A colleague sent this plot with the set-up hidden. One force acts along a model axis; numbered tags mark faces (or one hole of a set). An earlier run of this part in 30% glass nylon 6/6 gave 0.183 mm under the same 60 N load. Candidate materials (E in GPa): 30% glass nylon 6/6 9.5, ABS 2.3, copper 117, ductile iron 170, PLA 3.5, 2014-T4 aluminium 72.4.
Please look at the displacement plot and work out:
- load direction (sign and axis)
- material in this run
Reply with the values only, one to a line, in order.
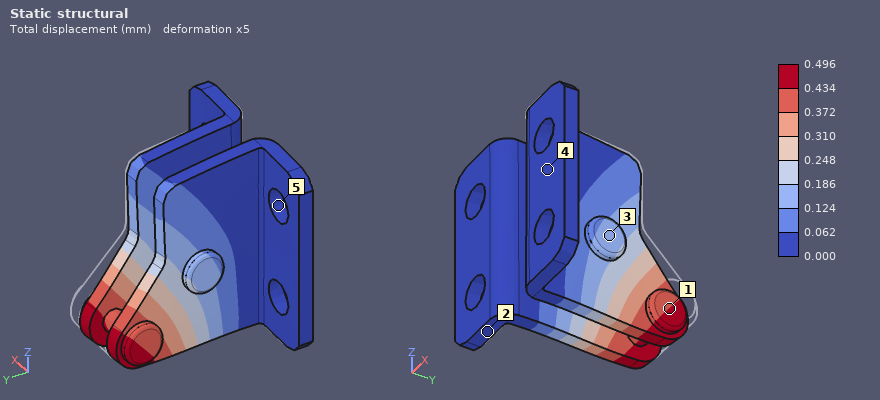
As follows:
-X
PLA
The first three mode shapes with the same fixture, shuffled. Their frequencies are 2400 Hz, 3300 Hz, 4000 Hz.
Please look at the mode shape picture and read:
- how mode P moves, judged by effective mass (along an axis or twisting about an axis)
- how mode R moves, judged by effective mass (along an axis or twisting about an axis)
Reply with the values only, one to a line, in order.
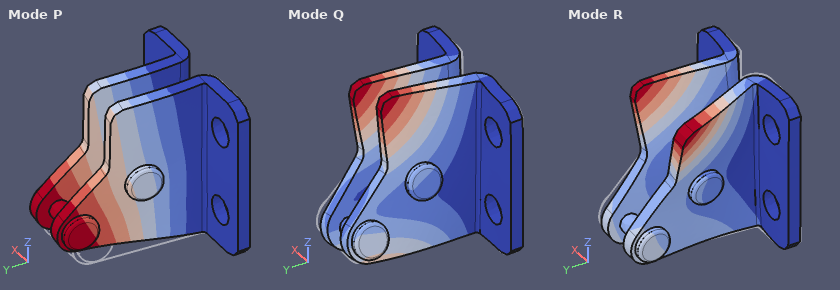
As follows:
along X
along Z
